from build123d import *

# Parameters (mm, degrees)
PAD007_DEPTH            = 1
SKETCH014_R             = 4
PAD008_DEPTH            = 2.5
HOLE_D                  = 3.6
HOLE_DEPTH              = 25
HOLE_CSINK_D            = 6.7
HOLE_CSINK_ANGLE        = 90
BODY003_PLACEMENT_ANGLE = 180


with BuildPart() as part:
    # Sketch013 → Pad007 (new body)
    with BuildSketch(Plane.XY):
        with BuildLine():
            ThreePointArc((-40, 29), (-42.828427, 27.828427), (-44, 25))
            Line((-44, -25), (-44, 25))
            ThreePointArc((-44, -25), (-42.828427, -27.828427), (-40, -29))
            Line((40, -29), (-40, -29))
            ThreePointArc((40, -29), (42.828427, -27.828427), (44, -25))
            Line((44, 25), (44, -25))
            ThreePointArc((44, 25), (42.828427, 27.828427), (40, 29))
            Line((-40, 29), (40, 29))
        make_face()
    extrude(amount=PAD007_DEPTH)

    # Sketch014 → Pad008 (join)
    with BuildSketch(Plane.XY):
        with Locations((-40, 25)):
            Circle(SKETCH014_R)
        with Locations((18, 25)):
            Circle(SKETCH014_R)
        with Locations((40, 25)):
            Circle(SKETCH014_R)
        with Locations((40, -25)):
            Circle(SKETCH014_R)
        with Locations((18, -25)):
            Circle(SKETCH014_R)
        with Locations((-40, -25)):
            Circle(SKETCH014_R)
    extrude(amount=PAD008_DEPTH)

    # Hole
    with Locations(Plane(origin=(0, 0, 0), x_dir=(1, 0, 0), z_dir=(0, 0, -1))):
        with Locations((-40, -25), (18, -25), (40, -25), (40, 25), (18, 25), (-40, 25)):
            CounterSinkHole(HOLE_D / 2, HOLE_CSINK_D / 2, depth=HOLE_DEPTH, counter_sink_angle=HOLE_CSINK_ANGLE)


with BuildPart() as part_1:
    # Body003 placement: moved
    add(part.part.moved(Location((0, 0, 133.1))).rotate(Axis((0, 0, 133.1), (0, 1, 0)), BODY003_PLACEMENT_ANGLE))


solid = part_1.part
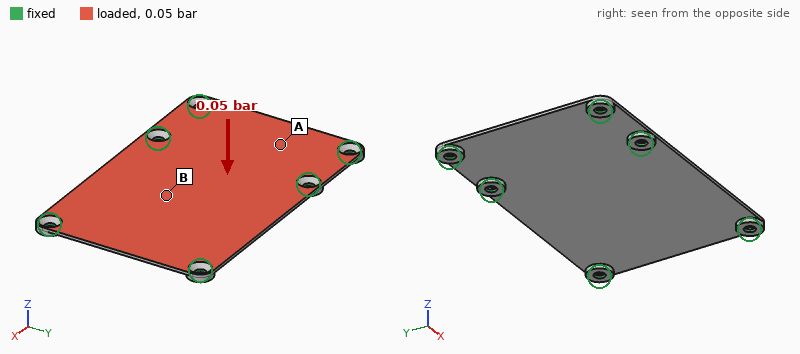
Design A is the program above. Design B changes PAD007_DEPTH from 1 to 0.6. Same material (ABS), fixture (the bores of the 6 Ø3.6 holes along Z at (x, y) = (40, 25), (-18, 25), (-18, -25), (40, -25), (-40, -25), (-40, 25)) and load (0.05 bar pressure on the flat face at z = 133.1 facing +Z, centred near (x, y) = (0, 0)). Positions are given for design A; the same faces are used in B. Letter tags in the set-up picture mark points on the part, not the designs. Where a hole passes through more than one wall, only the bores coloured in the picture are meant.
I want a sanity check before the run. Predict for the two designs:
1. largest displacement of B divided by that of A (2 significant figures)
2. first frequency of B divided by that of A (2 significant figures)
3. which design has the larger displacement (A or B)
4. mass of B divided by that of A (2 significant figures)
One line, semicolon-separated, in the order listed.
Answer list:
4.2; 0.63; B; 0.64
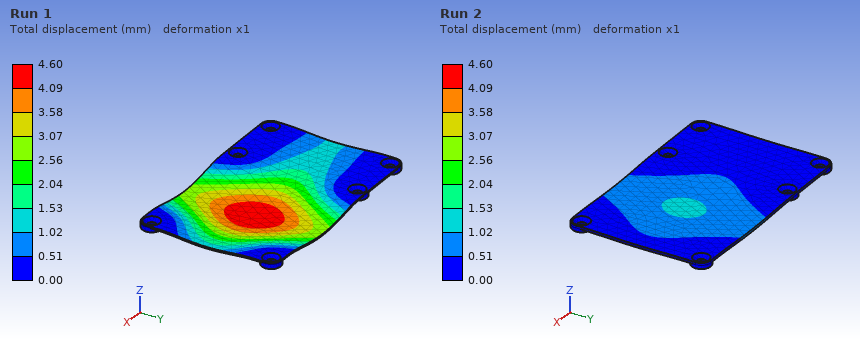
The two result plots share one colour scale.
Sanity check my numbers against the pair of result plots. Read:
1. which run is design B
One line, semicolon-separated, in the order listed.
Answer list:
Run 1
